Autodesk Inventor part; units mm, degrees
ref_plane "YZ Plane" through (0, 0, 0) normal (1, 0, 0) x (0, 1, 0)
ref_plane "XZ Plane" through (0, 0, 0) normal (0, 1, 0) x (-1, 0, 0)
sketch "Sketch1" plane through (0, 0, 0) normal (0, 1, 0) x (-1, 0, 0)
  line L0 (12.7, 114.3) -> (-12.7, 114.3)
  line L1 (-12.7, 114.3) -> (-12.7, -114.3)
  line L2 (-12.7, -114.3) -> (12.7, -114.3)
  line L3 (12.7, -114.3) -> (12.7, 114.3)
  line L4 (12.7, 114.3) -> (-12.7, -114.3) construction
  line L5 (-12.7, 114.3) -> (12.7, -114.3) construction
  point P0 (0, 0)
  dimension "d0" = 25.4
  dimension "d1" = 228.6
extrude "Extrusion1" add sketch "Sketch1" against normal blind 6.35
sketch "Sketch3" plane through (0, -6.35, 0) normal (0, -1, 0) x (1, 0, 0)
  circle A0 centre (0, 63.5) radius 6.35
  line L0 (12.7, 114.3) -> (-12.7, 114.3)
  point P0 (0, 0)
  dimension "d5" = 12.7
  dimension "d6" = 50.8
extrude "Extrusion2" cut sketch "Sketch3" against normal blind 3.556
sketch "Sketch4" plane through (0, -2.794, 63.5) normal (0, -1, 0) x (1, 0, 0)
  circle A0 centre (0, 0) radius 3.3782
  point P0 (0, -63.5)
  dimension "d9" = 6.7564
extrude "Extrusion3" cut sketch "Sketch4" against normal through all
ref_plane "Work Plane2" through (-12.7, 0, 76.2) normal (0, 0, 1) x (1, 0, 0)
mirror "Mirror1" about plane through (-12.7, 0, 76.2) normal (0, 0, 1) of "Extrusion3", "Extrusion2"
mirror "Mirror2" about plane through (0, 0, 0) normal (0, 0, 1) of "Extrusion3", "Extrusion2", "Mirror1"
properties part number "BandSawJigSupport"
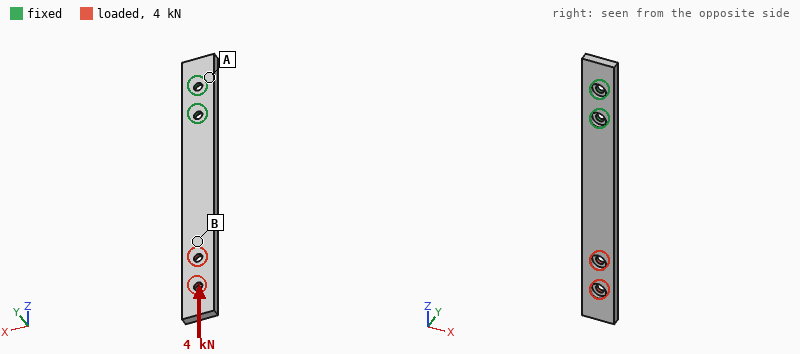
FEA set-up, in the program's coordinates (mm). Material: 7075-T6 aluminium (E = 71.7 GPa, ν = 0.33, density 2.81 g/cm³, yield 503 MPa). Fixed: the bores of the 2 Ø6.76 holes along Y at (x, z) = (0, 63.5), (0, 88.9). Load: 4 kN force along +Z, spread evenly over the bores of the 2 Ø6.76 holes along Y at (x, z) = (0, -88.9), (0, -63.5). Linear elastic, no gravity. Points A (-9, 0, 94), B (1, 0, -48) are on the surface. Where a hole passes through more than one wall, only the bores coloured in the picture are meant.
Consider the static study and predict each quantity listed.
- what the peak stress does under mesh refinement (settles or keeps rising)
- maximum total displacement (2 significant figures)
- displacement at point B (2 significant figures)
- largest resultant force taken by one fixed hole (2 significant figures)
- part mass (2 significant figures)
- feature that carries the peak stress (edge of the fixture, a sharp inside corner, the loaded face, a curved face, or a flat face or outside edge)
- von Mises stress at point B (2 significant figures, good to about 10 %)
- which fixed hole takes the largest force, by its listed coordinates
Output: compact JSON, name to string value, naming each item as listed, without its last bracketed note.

{"what the peak stress does under mesh refinement": "keeps rising", "maximum total displacement": "2.7 mm", "displacement at point B": "1.1 mm", "largest resultant force taken by one fixed hole": "3.4 kN", "part mass": "97 g", "feature that carries the peak stress": "edge of the fixture", "von Mises stress at point B": "64 MPa", "which fixed hole takes the largest force, by its listed coordinates": "(0, 63.5)"}
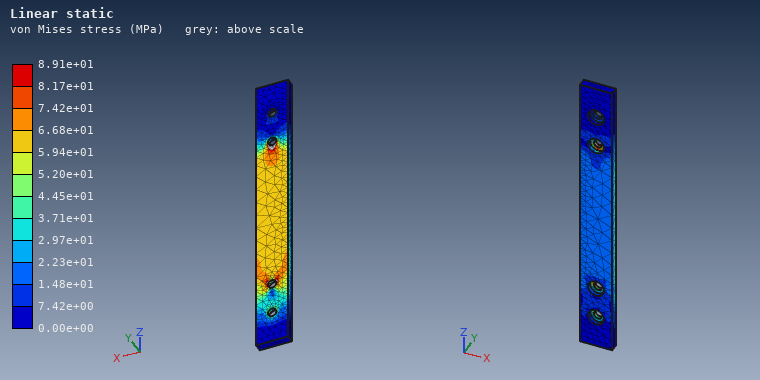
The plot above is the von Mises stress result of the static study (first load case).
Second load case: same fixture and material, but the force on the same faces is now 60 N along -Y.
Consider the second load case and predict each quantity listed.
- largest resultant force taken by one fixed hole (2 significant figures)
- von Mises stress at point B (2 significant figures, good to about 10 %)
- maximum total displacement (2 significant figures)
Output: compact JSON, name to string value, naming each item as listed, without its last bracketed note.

{"largest resultant force taken by one fixed hole": "580 N", "von Mises stress at point B": "10.0 MPa", "maximum total displacement": "2.2 mm"}
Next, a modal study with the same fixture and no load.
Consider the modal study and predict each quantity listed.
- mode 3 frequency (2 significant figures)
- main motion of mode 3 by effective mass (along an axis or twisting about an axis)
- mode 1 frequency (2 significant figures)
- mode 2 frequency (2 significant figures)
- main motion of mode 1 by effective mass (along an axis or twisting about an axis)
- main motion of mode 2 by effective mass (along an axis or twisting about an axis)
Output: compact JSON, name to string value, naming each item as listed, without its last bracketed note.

{"mode 3 frequency": "950 Hz", "main motion of mode 3 by effective mass": "along Y", "mode 1 frequency": "160 Hz", "mode 2 frequency": "590 Hz", "main motion of mode 1 by effective mass": "along Y", "main motion of mode 2 by effective mass": "along X"}
